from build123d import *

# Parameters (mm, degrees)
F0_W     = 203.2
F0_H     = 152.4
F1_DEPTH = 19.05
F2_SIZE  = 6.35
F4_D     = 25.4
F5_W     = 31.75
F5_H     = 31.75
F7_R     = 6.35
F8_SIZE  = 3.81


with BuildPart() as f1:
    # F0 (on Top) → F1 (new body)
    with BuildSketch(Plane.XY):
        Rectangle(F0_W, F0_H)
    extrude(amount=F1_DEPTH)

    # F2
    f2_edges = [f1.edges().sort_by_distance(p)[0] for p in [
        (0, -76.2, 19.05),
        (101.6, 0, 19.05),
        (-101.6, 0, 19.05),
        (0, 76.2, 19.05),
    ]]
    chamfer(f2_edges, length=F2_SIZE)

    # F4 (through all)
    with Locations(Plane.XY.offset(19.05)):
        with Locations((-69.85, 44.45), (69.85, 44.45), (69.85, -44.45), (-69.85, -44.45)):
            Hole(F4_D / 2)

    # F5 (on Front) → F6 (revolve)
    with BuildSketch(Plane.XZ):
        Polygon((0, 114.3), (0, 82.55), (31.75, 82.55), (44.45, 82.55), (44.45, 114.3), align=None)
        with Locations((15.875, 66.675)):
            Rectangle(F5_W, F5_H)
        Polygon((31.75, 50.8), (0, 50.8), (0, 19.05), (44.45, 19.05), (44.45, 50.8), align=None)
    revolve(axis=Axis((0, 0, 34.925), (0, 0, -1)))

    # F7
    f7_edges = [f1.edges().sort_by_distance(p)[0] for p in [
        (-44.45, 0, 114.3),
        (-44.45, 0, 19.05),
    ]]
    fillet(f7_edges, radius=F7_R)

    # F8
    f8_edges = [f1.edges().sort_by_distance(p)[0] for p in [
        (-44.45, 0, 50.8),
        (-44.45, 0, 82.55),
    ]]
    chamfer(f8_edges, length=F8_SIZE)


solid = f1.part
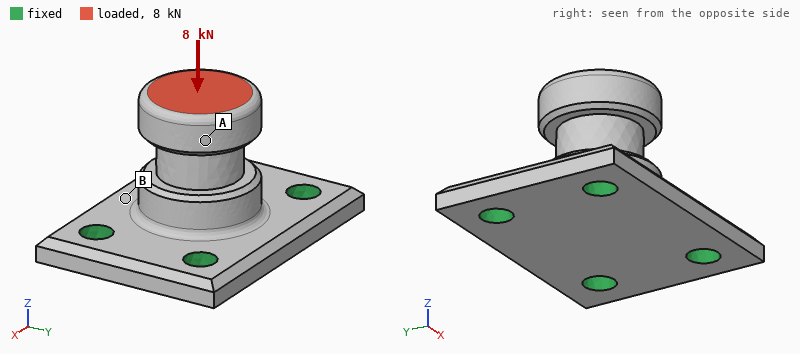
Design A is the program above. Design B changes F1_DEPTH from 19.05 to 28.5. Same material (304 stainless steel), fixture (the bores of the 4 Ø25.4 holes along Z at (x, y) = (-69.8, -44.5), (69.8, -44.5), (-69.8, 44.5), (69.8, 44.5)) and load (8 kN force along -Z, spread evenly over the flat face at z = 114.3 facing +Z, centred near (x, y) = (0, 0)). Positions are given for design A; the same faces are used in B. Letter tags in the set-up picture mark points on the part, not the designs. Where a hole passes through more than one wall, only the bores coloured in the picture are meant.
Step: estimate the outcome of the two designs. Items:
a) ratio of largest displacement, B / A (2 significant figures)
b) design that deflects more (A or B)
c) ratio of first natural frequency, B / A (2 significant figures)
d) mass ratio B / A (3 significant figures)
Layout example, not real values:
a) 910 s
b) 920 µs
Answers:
a) 0.64
b) A
c) 1.4
d) 1.21
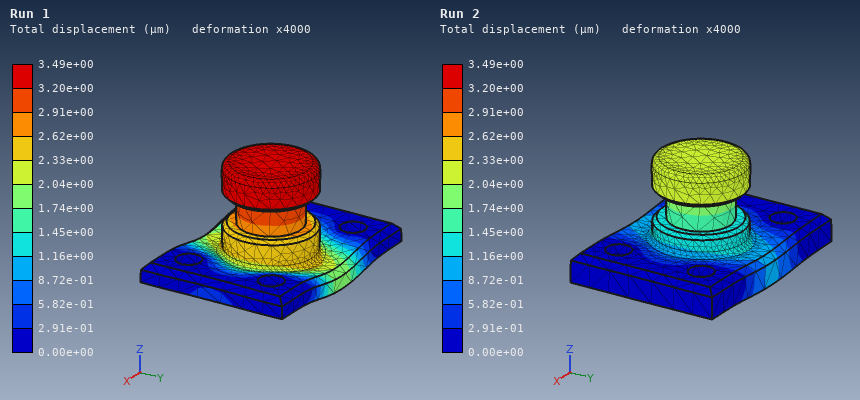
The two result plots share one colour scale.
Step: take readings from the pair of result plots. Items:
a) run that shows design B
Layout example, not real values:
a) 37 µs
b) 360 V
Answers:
a) Run 2
